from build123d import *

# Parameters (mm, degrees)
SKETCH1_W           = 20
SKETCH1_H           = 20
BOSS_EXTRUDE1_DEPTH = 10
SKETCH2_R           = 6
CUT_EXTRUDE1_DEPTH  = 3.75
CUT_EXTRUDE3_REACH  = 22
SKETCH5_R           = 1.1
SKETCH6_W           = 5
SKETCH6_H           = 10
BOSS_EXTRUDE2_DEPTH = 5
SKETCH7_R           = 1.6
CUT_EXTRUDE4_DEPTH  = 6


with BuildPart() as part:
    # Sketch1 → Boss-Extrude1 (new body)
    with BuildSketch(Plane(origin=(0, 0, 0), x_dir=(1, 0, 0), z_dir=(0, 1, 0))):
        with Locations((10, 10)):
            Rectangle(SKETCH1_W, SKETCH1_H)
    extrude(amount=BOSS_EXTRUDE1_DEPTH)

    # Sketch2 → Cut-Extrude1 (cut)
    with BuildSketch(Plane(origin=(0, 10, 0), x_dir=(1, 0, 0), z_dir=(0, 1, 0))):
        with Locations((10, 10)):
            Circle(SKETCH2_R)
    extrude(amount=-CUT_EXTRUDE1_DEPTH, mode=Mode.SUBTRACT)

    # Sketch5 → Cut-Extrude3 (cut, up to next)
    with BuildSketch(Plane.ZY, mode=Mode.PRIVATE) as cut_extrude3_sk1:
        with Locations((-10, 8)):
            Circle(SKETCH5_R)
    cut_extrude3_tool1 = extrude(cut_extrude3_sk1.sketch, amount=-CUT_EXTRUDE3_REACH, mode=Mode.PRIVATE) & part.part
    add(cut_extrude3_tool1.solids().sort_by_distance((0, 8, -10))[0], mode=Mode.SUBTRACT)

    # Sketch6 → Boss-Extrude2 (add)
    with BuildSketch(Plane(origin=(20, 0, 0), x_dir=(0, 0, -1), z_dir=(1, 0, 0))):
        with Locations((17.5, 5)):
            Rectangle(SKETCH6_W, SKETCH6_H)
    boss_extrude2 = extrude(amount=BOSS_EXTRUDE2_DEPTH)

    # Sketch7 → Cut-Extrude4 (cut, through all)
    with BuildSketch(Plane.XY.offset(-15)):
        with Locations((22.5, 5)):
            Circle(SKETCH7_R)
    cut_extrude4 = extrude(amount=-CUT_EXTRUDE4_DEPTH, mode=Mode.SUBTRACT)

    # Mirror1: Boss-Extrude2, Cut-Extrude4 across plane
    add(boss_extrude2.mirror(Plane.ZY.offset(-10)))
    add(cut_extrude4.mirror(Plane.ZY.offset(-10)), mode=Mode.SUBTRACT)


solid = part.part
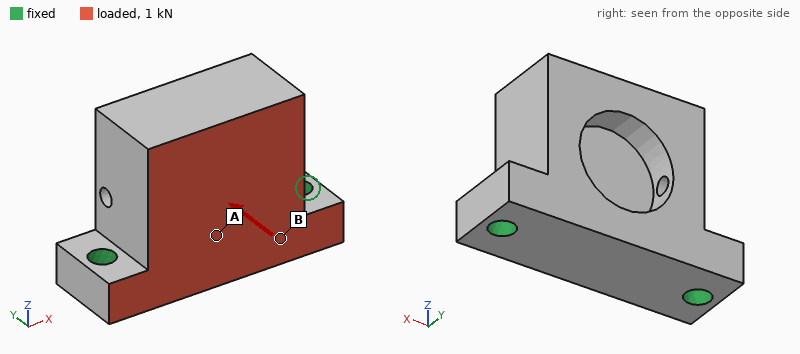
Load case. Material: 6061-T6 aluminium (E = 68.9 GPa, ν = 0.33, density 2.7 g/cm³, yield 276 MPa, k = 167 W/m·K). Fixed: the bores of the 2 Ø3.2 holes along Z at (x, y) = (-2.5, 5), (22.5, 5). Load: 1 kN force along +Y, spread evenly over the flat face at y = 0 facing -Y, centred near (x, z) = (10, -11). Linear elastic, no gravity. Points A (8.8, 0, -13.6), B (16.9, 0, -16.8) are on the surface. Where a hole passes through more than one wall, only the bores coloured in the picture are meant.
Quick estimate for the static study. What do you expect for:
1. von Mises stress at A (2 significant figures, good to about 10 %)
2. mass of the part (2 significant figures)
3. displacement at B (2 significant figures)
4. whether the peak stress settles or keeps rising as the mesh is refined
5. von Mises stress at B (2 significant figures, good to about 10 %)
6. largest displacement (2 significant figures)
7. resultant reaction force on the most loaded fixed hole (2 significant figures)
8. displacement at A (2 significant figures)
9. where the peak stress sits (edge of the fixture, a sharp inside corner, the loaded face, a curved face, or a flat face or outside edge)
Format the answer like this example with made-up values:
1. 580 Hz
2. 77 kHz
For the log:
1. 11 MPa
2. 11 g
3. 8.4 µm
4. keeps rising
5. 22 MPa
6. 37 µm
7. 500 N
8. 13 µm
9. edge of the fixture
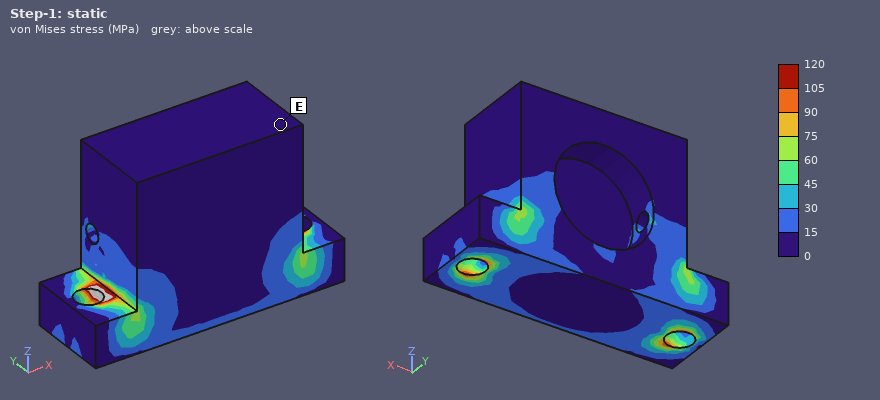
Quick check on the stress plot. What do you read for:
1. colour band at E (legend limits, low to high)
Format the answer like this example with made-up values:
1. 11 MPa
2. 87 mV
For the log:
1. 0 to 15 MPa
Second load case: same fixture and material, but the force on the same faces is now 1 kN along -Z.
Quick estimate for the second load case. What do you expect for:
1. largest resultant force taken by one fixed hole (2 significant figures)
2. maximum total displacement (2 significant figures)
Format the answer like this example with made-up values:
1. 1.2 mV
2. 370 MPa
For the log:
1. 520 N
2. 25 µm
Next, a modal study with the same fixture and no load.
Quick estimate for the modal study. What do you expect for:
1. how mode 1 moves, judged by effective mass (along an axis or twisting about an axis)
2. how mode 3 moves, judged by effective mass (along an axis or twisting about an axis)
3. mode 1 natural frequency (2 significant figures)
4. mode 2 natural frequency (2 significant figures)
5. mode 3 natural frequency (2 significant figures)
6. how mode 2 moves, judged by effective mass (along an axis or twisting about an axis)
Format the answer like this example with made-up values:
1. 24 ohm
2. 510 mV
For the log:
1. along Y
2. along X
3. 9500 Hz
4. 23 kHz
5. 28 kHz
6. along X
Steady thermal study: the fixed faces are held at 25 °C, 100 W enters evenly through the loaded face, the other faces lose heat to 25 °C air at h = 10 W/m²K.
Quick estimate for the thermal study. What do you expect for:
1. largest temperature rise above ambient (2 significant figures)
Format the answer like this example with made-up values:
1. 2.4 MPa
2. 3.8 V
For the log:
1. 51 K
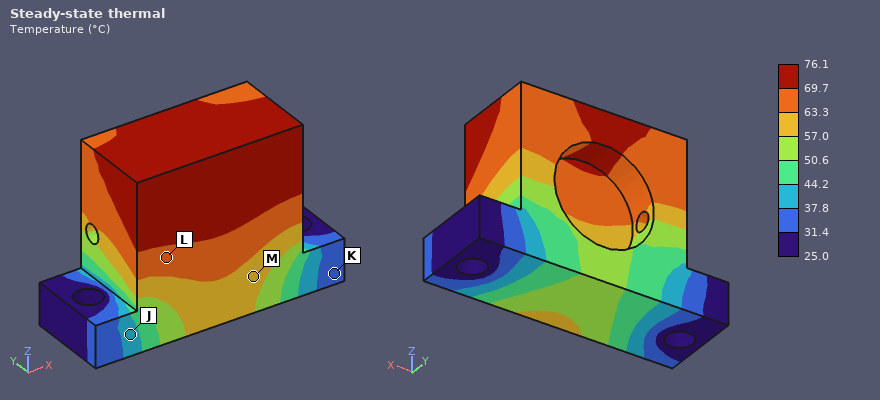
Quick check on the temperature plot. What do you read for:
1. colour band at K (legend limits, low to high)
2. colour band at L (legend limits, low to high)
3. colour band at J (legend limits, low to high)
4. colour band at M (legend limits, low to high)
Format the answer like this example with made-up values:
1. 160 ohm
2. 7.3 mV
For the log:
1. 31.4 to 37.8 °C
2. 63.3 to 69.7 °C
3. 37.8 to 44.2 °C
4. 57.0 to 63.3 °C
